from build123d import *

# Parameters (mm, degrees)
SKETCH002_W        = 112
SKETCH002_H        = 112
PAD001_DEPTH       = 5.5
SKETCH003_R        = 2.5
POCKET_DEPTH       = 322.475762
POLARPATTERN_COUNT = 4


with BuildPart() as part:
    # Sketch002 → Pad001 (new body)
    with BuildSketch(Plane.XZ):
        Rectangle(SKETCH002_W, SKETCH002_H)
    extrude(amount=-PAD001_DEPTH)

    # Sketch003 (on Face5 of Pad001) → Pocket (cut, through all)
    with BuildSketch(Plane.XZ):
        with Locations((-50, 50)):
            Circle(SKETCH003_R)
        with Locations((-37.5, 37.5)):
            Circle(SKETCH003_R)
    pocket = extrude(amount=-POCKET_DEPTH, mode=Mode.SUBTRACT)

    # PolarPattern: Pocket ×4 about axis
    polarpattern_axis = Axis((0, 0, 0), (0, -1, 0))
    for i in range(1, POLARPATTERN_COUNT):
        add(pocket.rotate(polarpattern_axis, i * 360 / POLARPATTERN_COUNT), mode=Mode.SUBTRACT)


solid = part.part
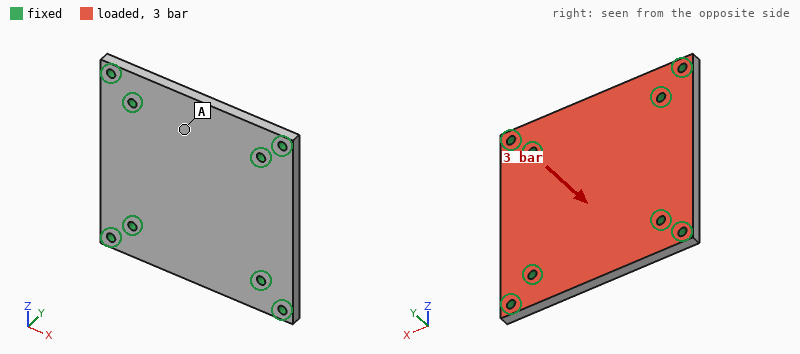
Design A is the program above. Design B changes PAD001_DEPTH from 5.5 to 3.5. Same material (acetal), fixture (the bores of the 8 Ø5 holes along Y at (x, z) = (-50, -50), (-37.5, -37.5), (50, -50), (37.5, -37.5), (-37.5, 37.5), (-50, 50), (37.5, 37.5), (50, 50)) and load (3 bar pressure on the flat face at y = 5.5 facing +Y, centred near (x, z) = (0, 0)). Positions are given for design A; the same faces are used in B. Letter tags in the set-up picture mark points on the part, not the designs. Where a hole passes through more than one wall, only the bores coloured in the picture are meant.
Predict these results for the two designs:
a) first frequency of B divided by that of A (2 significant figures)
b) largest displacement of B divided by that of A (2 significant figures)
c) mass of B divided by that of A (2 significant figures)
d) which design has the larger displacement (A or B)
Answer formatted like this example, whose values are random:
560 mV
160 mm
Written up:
0.66
3.6
0.64
B
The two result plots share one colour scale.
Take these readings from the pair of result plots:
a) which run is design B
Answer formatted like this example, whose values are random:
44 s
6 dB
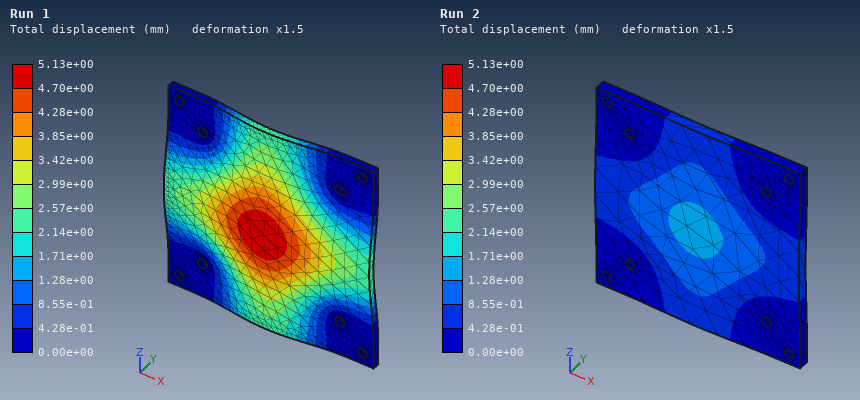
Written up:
Run 1
